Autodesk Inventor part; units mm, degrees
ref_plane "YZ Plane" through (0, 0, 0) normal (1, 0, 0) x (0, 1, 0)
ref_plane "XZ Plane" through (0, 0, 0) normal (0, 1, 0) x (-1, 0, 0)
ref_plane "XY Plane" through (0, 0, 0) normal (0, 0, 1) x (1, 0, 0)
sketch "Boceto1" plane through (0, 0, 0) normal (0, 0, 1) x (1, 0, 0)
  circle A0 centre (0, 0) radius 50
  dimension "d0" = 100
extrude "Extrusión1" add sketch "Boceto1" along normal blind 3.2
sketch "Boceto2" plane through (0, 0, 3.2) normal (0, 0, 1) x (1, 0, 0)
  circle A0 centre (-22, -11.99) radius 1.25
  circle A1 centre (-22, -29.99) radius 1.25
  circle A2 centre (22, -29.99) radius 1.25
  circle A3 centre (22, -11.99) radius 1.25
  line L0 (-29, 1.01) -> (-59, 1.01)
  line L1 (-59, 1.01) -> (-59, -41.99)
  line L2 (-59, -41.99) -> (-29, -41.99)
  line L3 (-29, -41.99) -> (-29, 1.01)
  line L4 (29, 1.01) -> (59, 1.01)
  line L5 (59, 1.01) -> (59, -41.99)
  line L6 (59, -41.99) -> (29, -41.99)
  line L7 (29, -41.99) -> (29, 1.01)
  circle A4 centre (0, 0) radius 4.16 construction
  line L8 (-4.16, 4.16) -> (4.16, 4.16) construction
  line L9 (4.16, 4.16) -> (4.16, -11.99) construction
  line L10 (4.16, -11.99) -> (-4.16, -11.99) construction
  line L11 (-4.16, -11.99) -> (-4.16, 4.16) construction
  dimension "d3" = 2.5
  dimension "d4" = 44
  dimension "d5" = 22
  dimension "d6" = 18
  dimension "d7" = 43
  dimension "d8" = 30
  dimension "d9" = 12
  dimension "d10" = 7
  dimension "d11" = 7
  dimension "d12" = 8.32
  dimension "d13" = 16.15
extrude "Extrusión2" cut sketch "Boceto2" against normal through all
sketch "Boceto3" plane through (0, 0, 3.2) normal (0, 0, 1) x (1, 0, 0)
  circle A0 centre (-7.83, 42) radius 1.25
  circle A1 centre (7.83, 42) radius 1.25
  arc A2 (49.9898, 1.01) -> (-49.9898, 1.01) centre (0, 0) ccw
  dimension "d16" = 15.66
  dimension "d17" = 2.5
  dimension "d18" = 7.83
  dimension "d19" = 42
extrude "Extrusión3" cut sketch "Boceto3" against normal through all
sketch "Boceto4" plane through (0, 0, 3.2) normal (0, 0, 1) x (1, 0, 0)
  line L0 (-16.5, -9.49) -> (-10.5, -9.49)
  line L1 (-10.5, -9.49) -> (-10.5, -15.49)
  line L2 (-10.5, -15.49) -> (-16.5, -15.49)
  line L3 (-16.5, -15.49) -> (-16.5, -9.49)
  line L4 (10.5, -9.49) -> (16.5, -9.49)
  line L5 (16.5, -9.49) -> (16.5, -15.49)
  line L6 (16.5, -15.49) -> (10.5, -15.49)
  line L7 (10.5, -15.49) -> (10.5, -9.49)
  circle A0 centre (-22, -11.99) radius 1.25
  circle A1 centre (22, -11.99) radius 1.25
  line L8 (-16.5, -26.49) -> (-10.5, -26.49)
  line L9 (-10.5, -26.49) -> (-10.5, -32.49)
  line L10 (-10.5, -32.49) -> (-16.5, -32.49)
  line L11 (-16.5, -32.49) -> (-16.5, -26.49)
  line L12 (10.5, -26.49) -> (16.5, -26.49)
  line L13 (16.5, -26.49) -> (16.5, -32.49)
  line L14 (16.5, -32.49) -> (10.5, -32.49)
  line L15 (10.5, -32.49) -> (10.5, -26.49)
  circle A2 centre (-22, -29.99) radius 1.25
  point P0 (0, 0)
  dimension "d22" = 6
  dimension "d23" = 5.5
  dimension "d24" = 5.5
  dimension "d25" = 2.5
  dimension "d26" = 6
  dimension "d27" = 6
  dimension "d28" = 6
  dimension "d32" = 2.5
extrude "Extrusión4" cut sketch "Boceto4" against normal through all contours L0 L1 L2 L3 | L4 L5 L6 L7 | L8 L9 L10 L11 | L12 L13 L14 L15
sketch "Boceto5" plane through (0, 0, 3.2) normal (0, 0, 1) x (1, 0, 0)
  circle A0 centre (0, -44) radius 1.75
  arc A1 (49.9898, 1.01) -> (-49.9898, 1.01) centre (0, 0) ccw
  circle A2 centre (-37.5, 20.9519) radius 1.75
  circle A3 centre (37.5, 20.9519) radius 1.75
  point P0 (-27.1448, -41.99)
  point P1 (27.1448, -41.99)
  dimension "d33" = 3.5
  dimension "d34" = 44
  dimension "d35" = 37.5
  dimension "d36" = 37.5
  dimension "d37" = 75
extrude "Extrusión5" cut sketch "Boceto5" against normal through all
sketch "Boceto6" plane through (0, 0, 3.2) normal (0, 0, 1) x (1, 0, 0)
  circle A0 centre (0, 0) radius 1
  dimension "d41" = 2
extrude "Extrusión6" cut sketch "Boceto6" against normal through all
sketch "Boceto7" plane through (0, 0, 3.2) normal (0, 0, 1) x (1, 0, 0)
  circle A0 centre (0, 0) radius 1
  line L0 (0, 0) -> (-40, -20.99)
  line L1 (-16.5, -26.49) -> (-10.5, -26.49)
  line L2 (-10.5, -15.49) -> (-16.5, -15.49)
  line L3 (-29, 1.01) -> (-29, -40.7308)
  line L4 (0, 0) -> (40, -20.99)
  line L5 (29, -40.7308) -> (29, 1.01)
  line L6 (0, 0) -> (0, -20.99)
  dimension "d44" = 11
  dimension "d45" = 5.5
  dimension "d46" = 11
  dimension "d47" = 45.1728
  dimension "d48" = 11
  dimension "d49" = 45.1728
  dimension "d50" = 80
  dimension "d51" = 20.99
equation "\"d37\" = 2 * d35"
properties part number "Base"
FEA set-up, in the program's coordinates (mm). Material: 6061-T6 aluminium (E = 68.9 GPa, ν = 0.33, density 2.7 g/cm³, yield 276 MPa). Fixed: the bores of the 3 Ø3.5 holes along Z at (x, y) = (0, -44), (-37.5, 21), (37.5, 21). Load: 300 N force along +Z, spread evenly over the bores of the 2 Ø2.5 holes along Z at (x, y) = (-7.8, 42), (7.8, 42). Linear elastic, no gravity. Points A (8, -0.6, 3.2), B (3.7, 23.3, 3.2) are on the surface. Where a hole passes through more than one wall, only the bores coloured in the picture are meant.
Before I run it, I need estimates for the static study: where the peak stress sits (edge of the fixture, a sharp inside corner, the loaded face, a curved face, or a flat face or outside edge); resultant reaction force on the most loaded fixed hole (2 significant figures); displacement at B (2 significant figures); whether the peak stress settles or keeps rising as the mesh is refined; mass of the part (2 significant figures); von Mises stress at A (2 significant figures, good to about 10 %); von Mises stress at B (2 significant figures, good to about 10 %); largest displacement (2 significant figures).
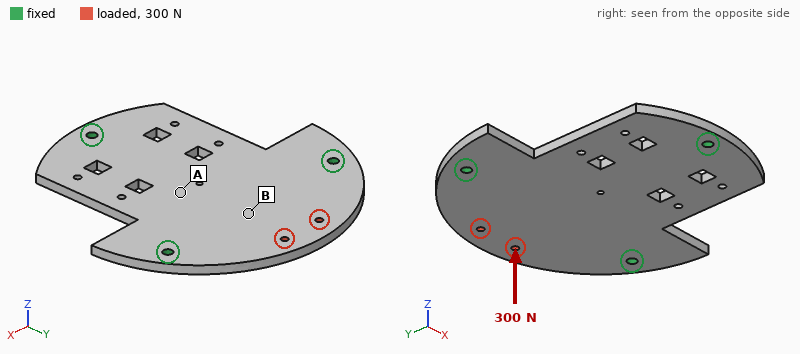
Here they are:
edge of the fixture
170 N
0.11 mm
keeps rising
55 g
16 MPa
37 MPa
0.37 mm
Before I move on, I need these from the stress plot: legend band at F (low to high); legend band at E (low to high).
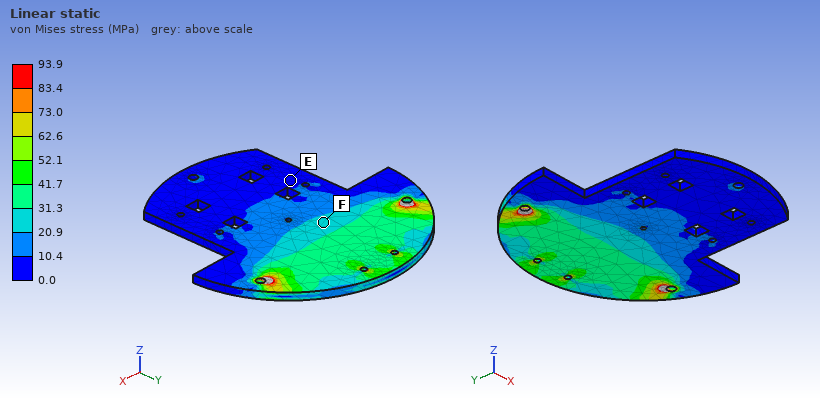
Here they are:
20.9 to 31.3 MPa
0.0 to 10.4 MPa
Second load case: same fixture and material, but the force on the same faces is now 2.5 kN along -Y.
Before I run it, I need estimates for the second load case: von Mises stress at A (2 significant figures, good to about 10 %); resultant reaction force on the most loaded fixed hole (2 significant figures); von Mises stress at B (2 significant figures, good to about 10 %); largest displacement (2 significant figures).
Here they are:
12 MPa
880 N
15 MPa
18 µm
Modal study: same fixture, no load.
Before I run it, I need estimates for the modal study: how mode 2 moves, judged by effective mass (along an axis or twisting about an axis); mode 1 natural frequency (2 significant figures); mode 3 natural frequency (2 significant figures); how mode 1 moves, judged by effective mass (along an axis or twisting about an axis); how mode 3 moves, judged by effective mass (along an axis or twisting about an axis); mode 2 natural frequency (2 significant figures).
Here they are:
along Z
2000 Hz
2900 Hz
along Z
twisting about Y
2500 Hz
